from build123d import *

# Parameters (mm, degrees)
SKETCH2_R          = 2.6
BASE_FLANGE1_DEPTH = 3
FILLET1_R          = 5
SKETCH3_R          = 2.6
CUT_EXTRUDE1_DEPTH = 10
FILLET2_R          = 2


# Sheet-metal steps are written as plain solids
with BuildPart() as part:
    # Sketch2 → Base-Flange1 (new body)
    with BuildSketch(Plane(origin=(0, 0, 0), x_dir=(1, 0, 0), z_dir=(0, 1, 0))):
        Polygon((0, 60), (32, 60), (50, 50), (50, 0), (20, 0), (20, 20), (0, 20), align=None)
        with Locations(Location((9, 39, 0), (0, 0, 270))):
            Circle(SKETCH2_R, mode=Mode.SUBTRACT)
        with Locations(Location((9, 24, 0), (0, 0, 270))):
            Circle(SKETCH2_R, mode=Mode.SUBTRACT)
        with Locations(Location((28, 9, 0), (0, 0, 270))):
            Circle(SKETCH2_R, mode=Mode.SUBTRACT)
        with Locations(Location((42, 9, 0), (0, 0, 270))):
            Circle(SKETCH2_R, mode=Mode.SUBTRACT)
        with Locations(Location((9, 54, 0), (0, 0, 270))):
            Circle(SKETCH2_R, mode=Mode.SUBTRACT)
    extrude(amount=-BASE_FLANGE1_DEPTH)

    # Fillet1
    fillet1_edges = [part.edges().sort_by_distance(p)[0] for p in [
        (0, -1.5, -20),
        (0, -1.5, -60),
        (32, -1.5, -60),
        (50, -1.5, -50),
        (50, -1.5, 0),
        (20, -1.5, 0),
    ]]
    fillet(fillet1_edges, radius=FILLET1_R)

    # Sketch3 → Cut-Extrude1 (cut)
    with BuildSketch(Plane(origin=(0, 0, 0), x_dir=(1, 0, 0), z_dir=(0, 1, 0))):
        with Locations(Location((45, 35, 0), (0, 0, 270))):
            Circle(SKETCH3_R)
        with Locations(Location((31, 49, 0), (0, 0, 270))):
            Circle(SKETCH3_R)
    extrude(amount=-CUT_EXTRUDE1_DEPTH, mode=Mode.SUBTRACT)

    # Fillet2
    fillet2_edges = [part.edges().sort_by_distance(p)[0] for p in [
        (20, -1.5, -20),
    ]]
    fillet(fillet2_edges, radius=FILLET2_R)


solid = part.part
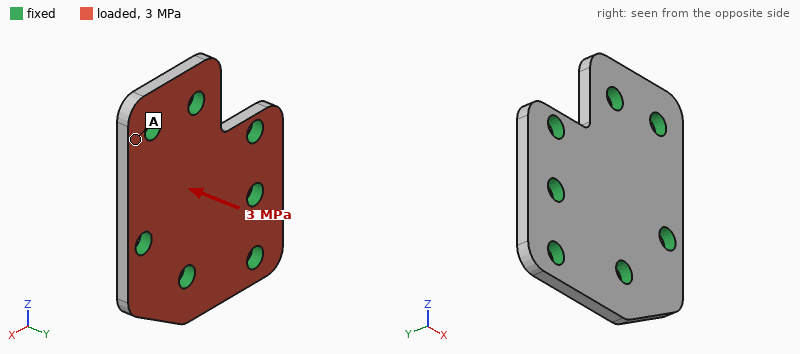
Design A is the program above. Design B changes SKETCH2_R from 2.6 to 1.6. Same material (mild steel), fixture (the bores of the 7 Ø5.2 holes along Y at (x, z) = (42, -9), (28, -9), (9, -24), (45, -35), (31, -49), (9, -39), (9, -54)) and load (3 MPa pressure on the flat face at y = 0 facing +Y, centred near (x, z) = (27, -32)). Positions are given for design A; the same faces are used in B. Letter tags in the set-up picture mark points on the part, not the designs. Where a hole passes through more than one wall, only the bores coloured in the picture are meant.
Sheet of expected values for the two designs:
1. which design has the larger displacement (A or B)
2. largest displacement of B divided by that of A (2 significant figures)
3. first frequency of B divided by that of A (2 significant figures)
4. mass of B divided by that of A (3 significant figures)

B
1.2
0.92
1.03
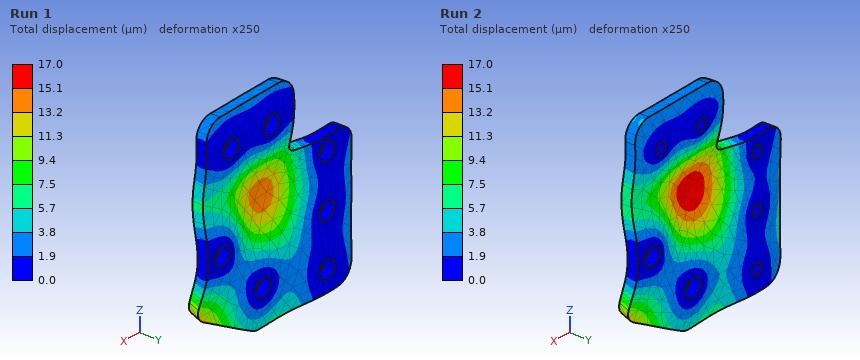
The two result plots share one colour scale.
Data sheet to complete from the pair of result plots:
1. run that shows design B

Run 2
